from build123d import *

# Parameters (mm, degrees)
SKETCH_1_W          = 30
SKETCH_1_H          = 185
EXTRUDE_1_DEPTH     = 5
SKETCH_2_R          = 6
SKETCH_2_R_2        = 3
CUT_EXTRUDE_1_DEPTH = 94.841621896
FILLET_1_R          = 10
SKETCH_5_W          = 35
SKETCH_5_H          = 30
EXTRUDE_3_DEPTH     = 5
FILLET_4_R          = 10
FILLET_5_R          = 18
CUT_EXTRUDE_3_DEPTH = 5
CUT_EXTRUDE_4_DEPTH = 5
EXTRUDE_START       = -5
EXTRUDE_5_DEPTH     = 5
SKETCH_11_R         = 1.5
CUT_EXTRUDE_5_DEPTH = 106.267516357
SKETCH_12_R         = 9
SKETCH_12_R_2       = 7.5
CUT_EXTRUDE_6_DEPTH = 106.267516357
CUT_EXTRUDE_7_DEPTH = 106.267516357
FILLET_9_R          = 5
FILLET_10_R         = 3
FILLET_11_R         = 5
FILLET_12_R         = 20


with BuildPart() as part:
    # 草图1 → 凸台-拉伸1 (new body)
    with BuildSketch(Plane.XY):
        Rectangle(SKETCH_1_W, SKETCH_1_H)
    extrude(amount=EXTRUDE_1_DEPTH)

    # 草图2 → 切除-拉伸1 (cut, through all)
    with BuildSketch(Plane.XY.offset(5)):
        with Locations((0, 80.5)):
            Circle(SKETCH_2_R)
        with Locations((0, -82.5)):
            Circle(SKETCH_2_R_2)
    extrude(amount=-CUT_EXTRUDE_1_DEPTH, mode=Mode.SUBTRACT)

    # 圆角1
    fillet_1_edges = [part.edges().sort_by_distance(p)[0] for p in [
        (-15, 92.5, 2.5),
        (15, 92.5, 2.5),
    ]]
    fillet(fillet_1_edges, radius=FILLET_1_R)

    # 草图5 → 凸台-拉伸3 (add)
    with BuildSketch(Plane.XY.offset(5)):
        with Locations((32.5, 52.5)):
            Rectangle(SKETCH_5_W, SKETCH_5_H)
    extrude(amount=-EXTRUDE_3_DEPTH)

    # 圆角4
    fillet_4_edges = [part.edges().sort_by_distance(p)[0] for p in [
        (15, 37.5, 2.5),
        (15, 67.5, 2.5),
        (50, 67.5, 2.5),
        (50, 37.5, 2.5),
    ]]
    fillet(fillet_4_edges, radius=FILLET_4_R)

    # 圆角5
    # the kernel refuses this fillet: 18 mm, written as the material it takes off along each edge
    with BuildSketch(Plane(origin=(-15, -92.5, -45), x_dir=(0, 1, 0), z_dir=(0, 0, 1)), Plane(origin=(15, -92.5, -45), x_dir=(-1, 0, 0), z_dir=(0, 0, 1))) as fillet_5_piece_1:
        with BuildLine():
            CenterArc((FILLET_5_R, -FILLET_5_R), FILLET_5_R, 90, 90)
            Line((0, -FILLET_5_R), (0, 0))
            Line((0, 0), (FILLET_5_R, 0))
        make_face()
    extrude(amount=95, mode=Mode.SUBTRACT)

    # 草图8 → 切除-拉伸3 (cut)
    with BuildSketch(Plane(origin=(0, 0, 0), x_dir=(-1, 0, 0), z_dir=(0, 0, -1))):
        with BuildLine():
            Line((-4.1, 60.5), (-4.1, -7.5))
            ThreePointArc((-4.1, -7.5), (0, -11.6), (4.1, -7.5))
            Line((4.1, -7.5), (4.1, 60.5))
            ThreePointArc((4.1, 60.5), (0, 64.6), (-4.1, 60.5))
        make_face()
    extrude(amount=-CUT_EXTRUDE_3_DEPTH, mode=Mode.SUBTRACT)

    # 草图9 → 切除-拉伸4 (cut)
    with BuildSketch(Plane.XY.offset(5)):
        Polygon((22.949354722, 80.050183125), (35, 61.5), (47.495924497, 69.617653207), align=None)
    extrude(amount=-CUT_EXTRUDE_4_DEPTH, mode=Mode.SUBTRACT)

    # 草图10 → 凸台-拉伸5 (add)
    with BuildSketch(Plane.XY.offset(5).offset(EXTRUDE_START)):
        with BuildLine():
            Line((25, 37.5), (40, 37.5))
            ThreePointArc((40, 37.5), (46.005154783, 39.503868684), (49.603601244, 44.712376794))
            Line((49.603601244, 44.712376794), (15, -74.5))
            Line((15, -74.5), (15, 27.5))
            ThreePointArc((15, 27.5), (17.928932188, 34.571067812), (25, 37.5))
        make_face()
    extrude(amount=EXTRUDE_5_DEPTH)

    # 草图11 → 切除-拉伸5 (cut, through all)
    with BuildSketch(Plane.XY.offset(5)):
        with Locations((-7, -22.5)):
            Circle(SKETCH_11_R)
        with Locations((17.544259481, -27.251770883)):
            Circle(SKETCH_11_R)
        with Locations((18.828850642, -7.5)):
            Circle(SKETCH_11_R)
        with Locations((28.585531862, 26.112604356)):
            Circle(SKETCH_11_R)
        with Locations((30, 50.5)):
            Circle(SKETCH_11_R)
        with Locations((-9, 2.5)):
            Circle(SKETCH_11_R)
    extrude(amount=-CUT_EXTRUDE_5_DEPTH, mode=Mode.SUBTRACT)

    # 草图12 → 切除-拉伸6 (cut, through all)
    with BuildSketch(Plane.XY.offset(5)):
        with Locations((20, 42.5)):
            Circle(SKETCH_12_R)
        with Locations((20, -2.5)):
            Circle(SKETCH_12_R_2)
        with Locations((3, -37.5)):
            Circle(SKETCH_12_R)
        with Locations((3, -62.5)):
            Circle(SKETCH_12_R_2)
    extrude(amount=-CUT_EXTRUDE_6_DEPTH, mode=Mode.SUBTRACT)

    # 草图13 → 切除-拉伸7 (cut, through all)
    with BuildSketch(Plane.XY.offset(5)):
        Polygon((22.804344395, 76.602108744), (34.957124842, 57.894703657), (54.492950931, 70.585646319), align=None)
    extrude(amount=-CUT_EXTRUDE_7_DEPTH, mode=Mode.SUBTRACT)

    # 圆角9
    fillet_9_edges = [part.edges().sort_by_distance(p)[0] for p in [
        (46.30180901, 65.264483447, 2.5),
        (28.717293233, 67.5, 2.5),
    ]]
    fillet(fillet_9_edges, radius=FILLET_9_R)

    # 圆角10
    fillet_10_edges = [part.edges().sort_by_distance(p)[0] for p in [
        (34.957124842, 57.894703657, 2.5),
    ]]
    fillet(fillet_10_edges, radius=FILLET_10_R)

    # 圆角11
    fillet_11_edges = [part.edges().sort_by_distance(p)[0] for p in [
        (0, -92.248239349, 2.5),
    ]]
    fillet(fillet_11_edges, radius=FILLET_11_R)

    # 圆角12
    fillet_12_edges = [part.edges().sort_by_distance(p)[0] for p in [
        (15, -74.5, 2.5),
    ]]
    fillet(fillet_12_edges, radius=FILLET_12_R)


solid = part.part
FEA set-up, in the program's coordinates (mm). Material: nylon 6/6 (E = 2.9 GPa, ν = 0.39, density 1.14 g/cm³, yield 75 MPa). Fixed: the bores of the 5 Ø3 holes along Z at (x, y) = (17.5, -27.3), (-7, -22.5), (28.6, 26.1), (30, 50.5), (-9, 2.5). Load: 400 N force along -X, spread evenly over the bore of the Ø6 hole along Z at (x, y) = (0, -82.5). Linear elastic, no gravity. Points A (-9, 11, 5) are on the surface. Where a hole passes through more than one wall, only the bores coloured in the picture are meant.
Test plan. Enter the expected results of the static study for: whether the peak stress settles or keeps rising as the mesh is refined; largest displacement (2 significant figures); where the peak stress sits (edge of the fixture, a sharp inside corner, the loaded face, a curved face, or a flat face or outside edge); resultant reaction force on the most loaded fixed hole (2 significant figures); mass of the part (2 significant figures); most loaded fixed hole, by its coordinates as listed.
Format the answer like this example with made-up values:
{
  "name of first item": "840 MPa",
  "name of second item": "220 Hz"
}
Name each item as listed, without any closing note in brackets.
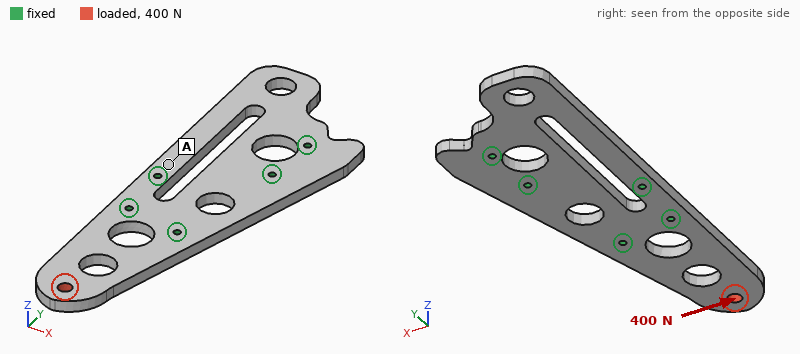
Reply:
{
  "whether the peak stress settles or keeps rising as the mesh is refined": "keeps rising",
  "largest displacement": "0.90 mm",
  "where the peak stress sits": "edge of the fixture",
  "resultant reaction force on the most loaded fixed hole": "710 N",
  "mass of the part": "37 g",
  "most loaded fixed hole, by its coordinates as listed": "(17.5, -27.3)"
}
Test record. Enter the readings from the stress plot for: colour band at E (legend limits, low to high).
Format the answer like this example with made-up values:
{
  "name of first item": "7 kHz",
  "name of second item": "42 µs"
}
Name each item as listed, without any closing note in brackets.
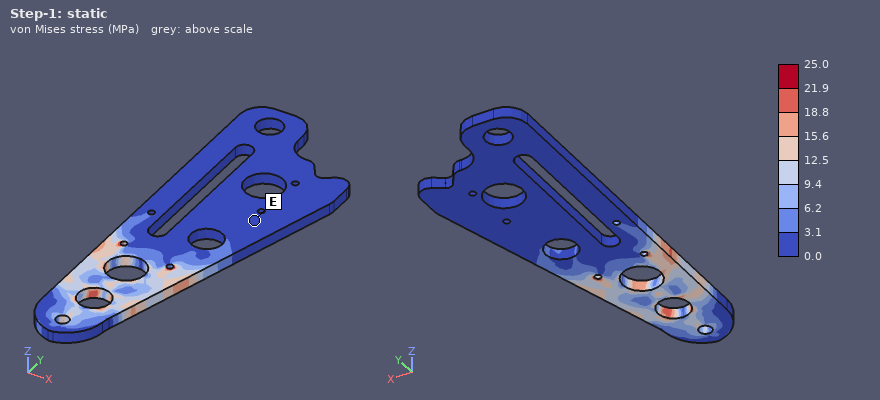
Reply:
{
  "colour band at E": "0.0 to 3.1 MPa"
}
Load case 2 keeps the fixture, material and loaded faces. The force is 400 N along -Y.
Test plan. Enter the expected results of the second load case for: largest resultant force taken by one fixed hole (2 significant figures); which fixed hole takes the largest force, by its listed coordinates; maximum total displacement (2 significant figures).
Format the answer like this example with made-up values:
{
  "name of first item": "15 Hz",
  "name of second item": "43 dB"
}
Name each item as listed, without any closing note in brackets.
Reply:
{
  "largest resultant force taken by one fixed hole": "230 N",
  "which fixed hole takes the largest force, by its listed coordinates": "(-7, -22.5)",
  "maximum total displacement": "0.13 mm"
}
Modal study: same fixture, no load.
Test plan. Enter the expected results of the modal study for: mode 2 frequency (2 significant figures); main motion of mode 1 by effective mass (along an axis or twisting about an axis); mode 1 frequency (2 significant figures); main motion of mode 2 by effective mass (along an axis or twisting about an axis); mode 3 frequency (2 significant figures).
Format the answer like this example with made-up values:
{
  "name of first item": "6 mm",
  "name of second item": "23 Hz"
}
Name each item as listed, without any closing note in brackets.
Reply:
{
  "mode 2 frequency": "400 Hz",
  "main motion of mode 1 by effective mass": "along Z",
  "mode 1 frequency": "310 Hz",
  "main motion of mode 2 by effective mass": "along Z",
  "mode 3 frequency": "1100 Hz"
}
